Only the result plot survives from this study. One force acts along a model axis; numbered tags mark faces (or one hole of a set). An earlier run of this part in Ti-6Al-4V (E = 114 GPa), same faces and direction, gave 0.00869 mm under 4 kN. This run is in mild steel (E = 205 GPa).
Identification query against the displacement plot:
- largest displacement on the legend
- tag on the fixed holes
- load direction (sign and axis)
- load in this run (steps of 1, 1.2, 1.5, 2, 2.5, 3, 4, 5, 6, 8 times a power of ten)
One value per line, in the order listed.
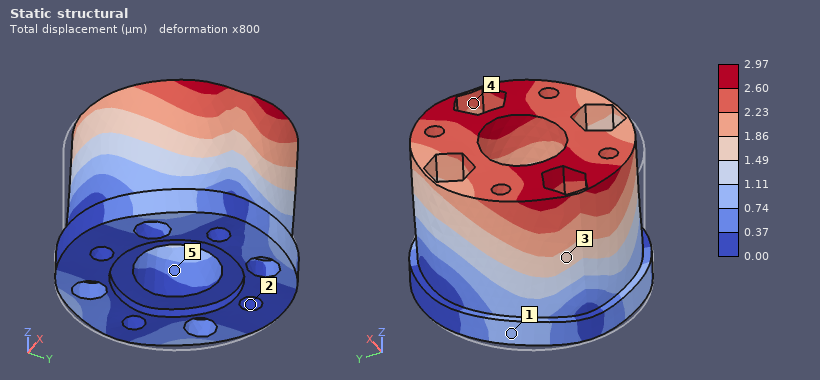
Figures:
2.97 µm
2
+X
2.5 kN
